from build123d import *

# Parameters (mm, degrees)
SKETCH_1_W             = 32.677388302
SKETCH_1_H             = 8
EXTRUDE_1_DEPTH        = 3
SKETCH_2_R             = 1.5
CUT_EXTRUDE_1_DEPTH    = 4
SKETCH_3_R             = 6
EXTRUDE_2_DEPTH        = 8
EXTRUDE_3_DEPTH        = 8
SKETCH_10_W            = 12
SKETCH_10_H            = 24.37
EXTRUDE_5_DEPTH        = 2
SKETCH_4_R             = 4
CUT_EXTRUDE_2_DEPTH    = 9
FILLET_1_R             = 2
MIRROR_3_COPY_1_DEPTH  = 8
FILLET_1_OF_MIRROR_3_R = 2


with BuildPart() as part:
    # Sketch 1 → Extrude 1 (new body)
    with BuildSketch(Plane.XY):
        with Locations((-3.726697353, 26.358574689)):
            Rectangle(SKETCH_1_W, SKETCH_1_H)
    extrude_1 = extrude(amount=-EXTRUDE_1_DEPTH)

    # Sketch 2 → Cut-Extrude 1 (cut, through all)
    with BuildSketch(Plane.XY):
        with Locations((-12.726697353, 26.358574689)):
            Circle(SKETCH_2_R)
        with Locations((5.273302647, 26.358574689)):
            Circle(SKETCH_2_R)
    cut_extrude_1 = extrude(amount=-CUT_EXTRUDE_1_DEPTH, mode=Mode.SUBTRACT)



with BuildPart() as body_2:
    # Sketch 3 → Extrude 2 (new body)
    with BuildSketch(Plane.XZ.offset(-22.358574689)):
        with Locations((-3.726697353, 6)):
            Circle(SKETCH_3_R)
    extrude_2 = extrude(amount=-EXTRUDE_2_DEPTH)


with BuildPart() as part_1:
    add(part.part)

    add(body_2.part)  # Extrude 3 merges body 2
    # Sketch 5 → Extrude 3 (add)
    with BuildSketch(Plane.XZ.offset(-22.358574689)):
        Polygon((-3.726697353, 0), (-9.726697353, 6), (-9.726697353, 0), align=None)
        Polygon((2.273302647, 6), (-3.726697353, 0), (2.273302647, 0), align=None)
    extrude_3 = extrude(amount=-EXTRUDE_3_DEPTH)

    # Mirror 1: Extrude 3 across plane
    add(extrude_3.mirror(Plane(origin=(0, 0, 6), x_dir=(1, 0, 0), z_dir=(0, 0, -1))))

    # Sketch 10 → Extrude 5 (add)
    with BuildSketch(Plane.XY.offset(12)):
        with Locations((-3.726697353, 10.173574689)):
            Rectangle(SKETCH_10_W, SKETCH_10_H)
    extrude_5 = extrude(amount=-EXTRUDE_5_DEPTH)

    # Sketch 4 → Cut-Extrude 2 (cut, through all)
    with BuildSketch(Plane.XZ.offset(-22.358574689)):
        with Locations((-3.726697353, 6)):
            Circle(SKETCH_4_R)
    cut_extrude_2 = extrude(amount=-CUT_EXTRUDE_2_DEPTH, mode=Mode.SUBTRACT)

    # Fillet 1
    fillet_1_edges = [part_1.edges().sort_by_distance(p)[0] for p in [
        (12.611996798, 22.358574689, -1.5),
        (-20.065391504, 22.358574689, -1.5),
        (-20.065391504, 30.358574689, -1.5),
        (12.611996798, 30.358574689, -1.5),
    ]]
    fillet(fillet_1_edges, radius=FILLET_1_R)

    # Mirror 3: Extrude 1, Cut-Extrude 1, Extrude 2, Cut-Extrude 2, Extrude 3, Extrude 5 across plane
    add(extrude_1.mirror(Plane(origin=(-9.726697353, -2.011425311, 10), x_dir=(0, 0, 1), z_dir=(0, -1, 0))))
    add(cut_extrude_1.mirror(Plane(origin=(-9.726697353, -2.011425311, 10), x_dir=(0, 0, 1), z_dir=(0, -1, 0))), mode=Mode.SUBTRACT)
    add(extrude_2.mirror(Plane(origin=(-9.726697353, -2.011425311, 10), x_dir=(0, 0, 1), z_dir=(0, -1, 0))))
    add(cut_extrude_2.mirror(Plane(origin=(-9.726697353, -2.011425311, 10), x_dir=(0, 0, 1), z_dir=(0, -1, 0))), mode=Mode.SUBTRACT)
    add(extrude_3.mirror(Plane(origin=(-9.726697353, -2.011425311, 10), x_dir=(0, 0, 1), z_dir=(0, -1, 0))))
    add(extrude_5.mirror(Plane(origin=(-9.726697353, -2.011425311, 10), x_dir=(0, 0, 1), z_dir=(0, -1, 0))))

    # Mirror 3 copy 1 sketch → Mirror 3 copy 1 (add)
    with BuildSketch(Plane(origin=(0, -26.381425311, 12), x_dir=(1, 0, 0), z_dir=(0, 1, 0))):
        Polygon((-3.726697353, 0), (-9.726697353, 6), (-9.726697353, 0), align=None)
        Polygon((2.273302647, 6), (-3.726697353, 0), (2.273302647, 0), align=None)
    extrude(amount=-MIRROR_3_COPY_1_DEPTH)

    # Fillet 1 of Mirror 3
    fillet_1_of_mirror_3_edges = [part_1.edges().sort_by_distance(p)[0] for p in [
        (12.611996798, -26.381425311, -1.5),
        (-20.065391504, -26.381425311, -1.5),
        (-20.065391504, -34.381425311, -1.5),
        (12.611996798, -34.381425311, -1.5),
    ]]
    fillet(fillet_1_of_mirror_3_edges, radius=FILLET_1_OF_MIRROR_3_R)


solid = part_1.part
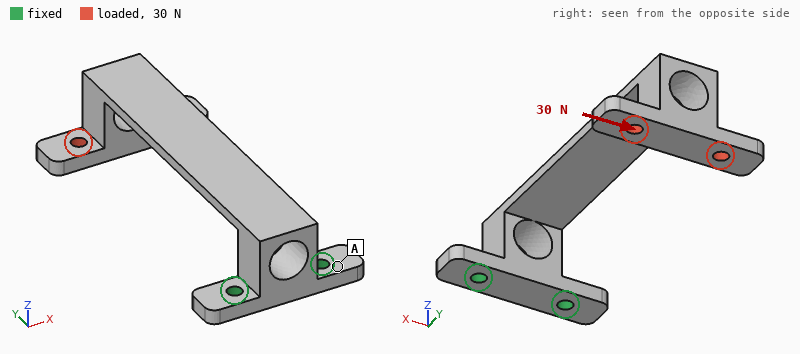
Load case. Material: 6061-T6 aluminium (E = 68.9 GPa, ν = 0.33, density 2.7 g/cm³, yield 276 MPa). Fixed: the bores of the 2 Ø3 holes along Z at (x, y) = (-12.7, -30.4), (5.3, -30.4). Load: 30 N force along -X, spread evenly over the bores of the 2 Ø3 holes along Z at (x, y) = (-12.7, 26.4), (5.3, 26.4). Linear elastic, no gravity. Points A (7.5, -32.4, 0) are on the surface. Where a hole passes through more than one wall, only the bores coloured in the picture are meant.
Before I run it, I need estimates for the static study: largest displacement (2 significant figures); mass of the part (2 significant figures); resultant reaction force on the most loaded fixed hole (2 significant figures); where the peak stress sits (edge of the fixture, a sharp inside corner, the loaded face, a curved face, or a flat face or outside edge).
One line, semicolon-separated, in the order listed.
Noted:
0.69 mm; 11 g; 100 N; a curved face
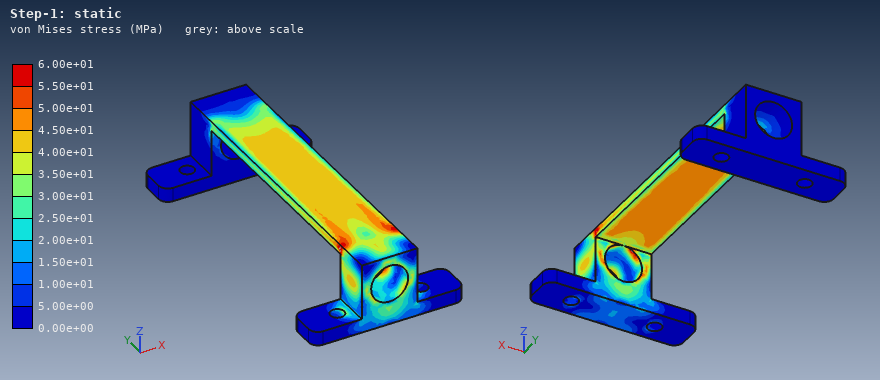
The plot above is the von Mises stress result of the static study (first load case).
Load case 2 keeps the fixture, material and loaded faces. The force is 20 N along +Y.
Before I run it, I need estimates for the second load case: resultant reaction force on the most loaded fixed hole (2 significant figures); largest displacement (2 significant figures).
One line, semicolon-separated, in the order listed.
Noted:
10 N; 0.82 mm
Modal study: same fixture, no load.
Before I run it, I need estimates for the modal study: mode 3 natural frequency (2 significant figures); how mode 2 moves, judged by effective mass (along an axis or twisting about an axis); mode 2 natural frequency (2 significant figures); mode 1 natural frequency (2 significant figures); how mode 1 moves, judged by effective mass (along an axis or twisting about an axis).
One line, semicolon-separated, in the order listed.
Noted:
1400 Hz; along X; 650 Hz; 230 Hz; along Z
